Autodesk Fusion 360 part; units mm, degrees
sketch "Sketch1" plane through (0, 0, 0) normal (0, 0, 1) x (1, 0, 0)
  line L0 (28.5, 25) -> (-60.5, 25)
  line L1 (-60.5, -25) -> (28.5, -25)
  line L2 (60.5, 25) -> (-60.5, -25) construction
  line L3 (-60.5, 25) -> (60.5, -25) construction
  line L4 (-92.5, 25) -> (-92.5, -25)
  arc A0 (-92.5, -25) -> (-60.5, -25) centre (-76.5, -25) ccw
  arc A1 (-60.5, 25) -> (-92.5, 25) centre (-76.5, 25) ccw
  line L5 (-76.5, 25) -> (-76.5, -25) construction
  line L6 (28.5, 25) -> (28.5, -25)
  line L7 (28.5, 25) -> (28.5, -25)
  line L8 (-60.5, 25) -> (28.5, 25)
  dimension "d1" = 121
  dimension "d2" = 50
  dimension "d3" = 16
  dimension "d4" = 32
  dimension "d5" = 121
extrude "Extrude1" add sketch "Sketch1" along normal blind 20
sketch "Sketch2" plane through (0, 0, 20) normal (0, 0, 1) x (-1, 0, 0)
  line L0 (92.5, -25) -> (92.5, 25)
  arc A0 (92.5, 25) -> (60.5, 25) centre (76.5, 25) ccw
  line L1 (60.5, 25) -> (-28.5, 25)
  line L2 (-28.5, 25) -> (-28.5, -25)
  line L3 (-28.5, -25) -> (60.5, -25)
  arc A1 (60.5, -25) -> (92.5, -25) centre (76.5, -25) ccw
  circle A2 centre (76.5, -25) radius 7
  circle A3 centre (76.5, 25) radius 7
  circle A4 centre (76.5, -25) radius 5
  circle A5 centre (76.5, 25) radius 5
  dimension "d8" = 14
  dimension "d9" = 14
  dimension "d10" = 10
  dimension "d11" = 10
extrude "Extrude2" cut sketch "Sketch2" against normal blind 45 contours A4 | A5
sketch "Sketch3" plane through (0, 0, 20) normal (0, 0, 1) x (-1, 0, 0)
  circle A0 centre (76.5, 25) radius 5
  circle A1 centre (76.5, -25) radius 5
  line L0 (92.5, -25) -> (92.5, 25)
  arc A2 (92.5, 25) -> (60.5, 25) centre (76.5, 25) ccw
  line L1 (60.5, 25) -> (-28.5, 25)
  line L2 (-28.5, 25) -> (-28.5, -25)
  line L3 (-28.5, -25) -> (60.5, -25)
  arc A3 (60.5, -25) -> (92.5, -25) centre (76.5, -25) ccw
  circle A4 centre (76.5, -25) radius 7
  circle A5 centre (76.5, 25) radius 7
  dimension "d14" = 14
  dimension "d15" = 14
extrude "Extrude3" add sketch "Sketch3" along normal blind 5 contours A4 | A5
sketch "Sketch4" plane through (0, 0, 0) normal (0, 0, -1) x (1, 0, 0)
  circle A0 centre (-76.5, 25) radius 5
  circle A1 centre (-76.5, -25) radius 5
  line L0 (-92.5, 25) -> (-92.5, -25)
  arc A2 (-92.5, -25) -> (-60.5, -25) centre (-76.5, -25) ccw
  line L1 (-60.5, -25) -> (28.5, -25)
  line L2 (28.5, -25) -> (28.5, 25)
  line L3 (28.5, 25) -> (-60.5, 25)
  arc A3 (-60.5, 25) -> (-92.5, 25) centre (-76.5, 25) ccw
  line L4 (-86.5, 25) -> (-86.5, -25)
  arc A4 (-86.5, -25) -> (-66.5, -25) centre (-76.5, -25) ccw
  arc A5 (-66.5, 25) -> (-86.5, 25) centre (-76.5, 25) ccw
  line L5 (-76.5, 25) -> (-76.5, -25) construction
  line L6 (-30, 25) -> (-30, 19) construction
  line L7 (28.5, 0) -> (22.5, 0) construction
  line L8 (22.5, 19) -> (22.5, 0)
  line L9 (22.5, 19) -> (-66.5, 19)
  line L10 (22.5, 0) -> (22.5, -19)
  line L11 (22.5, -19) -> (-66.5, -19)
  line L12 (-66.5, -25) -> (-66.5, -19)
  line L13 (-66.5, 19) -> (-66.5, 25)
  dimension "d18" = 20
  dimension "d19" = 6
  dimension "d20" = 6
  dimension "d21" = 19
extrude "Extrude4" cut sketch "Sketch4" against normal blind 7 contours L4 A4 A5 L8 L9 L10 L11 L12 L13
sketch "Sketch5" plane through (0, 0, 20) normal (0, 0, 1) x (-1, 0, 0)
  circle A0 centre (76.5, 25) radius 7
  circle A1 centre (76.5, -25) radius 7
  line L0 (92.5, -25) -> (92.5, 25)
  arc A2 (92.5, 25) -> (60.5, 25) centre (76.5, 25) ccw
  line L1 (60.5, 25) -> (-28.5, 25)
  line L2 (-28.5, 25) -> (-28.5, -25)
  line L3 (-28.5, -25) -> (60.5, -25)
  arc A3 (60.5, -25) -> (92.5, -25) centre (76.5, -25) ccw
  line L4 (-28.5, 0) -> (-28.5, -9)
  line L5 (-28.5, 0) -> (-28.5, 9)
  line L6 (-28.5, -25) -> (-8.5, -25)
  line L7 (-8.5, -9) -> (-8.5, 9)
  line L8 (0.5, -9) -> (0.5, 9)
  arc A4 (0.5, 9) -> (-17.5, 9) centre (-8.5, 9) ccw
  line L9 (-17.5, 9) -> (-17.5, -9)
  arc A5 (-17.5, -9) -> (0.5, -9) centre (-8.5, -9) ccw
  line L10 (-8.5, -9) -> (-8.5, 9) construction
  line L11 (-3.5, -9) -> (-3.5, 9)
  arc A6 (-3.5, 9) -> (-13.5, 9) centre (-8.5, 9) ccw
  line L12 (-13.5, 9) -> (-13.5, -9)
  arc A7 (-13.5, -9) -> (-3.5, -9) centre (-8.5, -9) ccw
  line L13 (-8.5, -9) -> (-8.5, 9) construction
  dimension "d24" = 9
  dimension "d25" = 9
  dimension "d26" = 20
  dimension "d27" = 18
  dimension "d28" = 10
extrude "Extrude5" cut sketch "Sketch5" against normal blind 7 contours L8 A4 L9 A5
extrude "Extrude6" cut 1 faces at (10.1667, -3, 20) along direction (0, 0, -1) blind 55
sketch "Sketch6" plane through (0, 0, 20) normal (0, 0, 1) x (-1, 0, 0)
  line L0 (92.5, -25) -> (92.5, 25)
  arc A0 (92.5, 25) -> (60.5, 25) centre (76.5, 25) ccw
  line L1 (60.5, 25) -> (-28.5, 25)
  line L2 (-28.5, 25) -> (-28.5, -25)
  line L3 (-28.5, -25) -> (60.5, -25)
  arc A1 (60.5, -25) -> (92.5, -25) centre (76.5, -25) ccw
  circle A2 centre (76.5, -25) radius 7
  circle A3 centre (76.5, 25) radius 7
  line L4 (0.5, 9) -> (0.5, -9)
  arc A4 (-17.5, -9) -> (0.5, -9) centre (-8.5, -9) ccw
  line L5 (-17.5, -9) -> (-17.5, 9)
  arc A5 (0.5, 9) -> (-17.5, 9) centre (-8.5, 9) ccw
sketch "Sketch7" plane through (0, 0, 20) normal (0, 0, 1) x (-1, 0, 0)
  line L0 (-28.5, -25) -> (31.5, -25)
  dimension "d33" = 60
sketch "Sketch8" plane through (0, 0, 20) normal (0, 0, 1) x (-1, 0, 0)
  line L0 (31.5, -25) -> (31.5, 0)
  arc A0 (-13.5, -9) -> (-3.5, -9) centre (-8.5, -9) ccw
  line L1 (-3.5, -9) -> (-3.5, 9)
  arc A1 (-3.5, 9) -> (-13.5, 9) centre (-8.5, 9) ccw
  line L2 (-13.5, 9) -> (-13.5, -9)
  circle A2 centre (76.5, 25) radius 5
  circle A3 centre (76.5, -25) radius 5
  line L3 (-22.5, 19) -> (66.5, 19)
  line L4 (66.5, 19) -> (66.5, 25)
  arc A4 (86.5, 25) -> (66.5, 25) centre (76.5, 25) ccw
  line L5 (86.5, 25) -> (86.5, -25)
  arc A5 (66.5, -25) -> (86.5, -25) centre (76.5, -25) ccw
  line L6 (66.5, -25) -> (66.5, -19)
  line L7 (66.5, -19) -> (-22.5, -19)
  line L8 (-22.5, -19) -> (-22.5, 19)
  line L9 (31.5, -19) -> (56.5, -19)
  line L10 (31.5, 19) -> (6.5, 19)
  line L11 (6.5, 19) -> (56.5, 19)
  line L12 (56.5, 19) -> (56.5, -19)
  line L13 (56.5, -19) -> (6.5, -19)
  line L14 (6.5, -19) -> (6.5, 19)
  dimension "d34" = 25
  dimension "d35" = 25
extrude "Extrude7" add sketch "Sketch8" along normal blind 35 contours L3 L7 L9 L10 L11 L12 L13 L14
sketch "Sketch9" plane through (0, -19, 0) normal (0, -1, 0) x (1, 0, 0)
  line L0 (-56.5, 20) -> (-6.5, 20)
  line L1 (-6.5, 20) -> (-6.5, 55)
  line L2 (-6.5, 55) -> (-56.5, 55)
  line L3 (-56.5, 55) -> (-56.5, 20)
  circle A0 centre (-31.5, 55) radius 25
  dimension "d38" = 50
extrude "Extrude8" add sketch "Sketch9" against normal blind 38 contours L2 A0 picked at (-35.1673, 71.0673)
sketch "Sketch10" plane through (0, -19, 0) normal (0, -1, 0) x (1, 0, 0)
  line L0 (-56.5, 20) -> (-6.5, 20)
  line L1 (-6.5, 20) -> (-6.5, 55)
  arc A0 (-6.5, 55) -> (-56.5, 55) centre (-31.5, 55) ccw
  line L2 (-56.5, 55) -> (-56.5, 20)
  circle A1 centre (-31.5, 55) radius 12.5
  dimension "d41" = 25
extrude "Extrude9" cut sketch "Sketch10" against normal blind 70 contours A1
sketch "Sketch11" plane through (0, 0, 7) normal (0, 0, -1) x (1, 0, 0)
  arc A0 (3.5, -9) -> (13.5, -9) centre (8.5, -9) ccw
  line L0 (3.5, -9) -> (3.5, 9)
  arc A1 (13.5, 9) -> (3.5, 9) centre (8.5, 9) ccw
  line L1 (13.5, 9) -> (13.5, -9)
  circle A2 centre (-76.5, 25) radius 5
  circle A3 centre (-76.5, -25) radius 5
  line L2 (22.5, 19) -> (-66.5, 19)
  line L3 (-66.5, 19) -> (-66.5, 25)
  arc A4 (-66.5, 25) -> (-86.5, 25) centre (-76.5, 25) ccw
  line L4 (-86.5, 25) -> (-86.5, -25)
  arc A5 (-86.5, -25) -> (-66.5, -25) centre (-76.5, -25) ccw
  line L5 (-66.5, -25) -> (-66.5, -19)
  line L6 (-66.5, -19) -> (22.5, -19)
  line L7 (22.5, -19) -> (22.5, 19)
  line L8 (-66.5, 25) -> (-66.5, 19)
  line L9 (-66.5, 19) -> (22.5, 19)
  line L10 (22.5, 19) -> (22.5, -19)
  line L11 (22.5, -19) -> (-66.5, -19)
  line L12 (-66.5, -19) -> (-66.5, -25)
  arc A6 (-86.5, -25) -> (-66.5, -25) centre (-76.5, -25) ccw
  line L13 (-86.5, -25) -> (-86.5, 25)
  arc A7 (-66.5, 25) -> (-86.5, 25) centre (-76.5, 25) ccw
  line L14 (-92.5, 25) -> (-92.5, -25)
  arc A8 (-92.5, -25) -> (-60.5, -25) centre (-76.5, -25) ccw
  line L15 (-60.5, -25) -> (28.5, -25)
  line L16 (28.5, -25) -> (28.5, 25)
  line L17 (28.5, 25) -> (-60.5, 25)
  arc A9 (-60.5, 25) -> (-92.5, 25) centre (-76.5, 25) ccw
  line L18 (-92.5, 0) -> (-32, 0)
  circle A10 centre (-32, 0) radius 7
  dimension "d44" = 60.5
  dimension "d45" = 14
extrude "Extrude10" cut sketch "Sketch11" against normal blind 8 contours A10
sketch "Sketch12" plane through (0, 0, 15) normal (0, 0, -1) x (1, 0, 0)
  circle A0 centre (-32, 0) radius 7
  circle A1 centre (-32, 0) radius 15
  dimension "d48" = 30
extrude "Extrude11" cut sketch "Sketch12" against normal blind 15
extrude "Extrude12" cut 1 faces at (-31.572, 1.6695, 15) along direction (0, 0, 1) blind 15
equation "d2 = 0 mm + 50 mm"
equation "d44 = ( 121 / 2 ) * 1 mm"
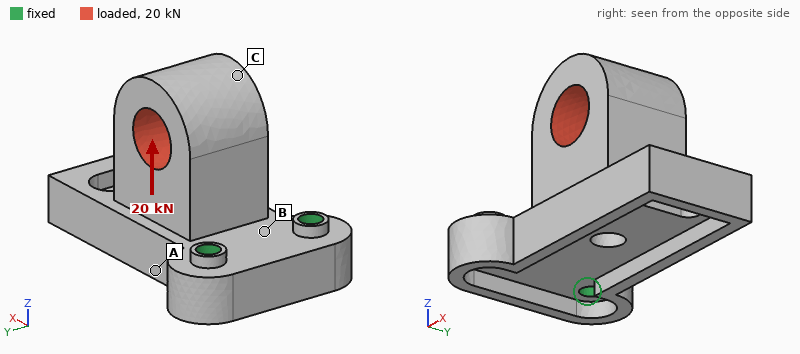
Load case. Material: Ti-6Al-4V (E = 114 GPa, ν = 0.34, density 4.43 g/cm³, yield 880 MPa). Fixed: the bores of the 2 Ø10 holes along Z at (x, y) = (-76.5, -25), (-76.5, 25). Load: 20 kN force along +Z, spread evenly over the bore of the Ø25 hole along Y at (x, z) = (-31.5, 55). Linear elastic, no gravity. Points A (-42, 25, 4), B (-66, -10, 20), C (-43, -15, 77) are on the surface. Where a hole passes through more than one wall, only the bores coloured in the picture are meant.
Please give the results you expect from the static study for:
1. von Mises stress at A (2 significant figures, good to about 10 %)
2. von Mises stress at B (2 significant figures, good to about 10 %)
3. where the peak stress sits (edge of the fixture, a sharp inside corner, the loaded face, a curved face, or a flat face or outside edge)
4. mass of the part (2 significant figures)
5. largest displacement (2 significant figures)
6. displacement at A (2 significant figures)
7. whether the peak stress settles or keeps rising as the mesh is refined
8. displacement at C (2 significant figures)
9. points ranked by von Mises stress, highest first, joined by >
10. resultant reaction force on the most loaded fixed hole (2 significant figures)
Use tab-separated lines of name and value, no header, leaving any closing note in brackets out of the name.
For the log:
von Mises stress at A	90 MPa
von Mises stress at B	270 MPa
where the peak stress sits	edge of the fixture
mass of the part	760 g
largest displacement	1.1 mm
displacement at A	0.29 mm
whether the peak stress settles or keeps rising as the mesh is refined	keeps rising
displacement at C	0.81 mm
points ranked by von Mises stress, highest first, joined by >	B > A > C
resultant reaction force on the most loaded fixed hole	10 kN
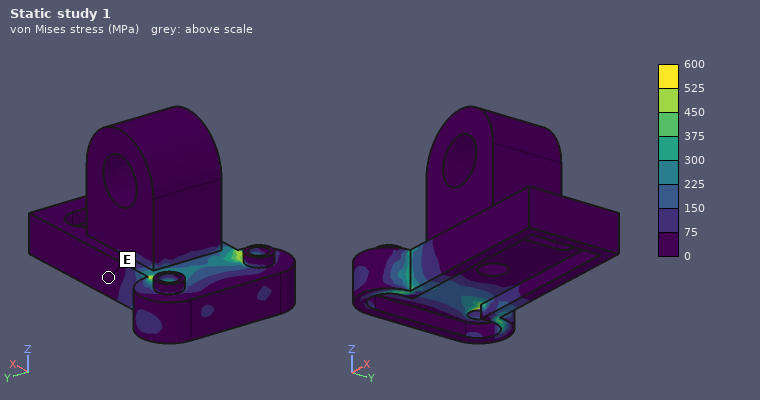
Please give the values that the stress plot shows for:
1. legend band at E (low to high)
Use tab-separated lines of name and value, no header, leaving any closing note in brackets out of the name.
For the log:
legend band at E	0 to 75 MPa
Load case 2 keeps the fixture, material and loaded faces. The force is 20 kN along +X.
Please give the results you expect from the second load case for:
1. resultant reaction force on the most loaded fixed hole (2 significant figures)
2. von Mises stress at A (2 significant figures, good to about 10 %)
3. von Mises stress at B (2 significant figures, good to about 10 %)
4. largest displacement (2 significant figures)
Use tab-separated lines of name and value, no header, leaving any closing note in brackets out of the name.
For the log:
resultant reaction force on the most loaded fixed hole	10 kN
von Mises stress at A	150 MPa
von Mises stress at B	360 MPa
largest displacement	1.4 mm
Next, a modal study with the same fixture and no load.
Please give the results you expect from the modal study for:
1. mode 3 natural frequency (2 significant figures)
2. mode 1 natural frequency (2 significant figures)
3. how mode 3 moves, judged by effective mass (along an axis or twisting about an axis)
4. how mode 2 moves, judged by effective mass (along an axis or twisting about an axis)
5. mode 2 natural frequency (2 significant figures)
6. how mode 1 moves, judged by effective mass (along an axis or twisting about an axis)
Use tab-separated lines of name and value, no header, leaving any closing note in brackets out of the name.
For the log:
mode 3 natural frequency	3300 Hz
mode 1 natural frequency	880 Hz
how mode 3 moves, judged by effective mass	along Y
how mode 2 moves, judged by effective mass	along Y
mode 2 natural frequency	2300 Hz
how mode 1 moves, judged by effective mass	along Z
